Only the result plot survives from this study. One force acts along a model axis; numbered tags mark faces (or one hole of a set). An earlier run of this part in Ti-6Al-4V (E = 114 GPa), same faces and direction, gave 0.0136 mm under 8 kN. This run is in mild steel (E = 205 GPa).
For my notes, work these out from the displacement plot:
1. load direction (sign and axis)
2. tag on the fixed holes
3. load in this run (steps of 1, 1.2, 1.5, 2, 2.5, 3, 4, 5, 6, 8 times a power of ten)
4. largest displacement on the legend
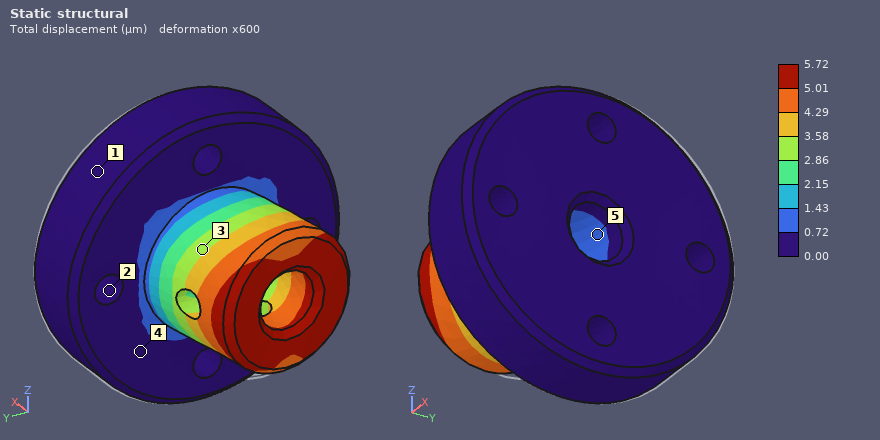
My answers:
-Y
2
6 kN
5.72 µm
